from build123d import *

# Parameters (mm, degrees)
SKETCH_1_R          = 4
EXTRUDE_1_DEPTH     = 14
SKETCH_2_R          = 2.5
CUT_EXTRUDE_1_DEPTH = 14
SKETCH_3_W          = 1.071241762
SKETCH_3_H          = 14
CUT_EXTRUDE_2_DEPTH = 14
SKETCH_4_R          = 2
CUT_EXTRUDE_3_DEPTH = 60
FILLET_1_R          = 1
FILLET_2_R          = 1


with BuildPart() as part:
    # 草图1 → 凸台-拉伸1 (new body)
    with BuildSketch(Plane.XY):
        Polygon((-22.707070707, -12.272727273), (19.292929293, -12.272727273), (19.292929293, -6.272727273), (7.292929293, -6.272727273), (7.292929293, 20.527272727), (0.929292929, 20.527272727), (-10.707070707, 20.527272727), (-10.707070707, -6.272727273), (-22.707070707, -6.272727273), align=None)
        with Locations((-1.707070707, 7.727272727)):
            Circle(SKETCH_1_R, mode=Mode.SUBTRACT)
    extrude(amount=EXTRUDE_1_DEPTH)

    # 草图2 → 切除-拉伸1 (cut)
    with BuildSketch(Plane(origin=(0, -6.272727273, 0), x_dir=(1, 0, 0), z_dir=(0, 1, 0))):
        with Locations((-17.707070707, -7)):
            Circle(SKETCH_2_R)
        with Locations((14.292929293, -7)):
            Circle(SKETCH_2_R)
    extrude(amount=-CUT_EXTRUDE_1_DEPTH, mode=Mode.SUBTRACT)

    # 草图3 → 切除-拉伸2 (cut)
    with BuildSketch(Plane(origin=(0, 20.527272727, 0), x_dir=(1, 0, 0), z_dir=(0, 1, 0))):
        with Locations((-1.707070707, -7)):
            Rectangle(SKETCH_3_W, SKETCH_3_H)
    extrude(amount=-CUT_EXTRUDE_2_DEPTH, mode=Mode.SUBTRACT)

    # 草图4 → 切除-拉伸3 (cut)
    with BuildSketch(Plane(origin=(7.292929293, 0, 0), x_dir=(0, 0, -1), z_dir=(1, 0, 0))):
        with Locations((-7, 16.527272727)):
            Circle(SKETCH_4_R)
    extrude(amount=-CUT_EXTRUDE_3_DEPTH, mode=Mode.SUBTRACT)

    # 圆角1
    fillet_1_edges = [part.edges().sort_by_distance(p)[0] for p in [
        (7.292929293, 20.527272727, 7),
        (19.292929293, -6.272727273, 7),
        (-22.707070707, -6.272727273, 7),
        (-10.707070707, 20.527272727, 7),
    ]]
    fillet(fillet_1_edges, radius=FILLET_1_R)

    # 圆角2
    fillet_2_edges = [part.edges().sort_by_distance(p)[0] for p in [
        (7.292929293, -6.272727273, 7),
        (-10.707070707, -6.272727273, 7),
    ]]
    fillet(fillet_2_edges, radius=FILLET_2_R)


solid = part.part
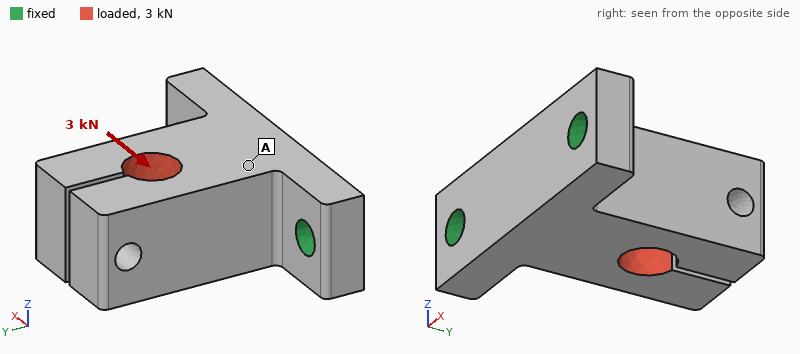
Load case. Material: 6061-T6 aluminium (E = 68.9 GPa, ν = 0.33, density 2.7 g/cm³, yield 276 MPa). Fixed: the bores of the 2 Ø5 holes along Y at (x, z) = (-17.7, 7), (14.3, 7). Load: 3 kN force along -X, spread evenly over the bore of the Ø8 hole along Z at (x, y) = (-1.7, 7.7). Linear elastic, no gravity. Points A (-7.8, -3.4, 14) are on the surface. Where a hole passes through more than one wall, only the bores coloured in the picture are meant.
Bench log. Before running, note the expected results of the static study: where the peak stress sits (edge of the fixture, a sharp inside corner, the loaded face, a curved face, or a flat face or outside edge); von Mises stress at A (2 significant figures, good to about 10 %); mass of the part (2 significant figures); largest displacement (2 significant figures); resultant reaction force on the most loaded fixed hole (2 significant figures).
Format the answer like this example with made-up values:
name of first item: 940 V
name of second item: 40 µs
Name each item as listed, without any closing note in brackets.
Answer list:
where the peak stress sits: a curved face
von Mises stress at A: 30 MPa
mass of the part: 24 g
largest displacement: 87 µm
resultant reaction force on the most loaded fixed hole: 2.5 kN
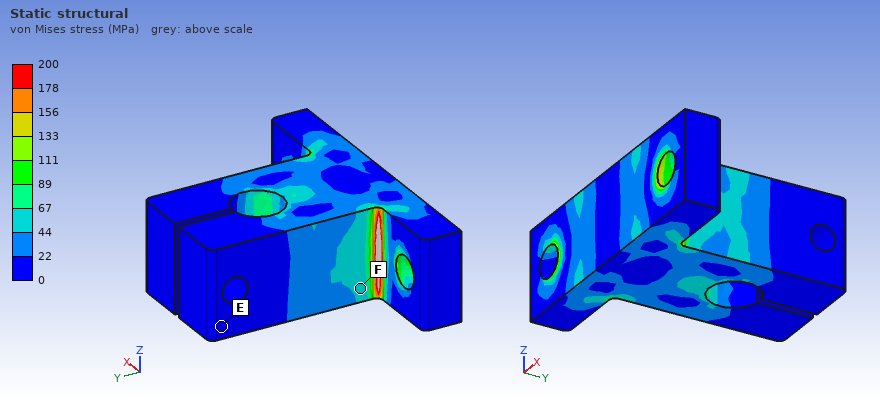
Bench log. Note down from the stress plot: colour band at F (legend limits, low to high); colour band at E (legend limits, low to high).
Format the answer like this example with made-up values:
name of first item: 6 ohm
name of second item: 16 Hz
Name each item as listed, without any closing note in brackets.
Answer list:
colour band at F: 44 to 67 MPa
colour band at E: 0 to 22 MPa
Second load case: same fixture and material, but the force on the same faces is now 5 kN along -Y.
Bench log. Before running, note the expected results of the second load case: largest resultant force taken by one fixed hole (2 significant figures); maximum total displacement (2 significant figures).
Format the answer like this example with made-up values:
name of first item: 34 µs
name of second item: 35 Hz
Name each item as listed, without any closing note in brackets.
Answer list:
largest resultant force taken by one fixed hole: 2.7 kN
maximum total displacement: 66 µm
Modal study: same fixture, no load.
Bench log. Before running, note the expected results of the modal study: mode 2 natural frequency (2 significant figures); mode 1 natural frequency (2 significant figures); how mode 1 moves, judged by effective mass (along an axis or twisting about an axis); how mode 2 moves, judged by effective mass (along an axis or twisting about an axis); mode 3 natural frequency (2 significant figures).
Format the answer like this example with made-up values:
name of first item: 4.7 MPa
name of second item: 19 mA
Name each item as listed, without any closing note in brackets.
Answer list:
mode 2 natural frequency: 8300 Hz
mode 1 natural frequency: 5000 Hz
how mode 1 moves, judged by effective mass: along Z
how mode 2 moves, judged by effective mass: along X
mode 3 natural frequency: 10 kHz
